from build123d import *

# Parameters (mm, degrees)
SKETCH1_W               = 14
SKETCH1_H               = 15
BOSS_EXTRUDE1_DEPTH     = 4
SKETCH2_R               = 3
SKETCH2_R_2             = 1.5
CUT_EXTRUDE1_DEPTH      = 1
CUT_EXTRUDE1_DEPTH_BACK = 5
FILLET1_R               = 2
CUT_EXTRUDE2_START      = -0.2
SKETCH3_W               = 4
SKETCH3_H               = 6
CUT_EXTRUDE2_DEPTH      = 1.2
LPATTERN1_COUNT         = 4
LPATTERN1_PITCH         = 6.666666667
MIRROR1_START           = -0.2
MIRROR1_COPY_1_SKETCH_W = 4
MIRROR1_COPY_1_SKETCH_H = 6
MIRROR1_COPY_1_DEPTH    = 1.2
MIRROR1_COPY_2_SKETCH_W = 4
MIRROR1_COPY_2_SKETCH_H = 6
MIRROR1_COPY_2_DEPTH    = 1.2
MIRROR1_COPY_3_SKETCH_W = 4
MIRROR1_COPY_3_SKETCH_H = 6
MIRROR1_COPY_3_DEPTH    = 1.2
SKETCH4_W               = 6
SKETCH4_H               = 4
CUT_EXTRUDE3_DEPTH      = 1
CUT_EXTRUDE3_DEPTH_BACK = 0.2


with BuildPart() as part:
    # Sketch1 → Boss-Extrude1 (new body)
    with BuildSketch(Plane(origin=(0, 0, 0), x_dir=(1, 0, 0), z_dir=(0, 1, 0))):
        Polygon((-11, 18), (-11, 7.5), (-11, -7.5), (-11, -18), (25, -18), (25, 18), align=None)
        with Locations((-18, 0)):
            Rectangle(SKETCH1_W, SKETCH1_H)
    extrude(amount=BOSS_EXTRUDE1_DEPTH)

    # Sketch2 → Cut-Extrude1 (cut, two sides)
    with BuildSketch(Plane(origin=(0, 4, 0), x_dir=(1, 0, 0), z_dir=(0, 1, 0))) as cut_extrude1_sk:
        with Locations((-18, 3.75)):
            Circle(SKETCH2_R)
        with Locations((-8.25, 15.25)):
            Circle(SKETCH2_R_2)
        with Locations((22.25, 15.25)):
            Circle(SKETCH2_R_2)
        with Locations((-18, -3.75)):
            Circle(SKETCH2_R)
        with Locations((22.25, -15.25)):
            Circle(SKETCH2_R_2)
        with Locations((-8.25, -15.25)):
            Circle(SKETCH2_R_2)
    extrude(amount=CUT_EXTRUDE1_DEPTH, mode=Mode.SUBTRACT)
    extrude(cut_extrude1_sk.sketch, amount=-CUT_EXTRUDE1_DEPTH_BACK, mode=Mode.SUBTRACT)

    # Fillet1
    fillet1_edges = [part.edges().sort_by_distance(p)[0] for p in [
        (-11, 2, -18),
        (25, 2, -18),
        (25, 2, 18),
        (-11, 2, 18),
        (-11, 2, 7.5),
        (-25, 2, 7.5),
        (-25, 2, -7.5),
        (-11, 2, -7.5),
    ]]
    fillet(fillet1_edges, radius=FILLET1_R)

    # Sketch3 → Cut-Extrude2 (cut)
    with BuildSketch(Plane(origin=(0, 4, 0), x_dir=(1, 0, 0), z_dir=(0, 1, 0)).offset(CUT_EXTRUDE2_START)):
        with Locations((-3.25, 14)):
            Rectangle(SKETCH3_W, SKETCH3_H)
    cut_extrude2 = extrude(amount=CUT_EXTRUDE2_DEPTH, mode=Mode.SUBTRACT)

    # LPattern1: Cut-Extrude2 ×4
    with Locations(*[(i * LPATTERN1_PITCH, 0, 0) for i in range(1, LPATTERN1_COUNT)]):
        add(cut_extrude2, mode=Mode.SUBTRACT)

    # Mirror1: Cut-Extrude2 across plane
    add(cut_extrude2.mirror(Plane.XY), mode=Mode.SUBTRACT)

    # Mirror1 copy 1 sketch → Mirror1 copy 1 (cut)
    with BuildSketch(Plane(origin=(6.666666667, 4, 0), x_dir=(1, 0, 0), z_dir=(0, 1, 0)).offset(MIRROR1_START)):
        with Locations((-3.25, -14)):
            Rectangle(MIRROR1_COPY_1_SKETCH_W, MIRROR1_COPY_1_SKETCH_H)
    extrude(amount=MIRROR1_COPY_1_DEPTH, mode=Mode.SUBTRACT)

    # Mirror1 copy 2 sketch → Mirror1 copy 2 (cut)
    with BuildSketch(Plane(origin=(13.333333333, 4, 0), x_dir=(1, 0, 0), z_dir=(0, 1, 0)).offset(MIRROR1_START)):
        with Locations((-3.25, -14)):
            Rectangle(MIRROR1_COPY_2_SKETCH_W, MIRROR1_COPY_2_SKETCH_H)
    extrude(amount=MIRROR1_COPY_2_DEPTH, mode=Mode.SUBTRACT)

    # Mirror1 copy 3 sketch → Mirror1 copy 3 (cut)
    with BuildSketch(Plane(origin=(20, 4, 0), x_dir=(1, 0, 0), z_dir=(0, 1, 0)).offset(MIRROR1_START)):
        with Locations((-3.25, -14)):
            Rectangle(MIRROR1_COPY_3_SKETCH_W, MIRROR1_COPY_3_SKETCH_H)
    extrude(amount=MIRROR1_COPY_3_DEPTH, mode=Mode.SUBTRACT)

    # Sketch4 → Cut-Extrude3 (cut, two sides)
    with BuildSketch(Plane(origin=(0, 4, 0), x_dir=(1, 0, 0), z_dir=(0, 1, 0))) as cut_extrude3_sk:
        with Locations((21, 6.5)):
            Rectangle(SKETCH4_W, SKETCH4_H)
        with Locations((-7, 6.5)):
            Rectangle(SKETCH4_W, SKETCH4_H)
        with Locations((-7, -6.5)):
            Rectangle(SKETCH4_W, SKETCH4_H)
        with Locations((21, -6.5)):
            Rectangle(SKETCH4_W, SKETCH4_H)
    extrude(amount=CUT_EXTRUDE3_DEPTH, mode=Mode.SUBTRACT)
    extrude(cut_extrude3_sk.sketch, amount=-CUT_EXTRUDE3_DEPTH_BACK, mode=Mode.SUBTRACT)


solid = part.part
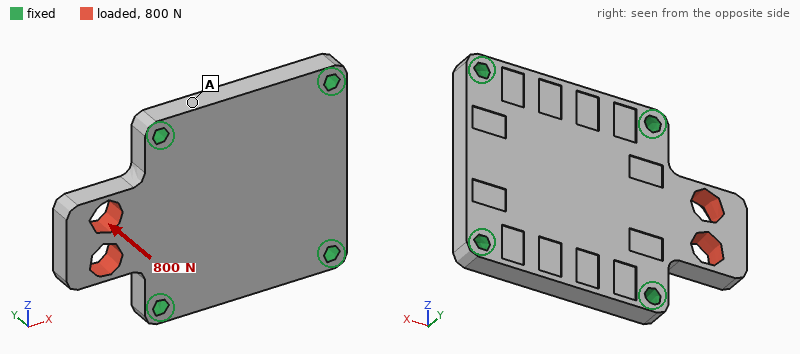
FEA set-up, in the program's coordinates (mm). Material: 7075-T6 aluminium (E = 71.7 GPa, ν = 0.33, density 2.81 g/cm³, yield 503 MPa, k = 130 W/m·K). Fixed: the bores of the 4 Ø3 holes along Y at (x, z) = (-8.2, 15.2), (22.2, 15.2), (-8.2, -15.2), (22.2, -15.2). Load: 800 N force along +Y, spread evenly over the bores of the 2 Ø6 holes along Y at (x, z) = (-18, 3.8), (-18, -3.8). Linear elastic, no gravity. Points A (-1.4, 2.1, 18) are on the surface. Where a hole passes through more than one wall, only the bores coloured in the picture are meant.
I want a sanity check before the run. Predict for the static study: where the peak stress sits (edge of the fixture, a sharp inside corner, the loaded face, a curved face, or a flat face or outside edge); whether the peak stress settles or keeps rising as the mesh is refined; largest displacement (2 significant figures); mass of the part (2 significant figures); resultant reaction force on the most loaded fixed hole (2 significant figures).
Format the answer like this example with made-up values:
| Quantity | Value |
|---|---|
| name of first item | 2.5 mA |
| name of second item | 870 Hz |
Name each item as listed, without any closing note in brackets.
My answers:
| Quantity | Value |
|---|---|
| where the peak stress sits | edge of the fixture |
| whether the peak stress settles or keeps rising as the mesh is refined | keeps rising |
| largest displacement | 0.26 mm |
| mass of the part | 16 g |
| resultant reaction force on the most loaded fixed hole | 500 N |
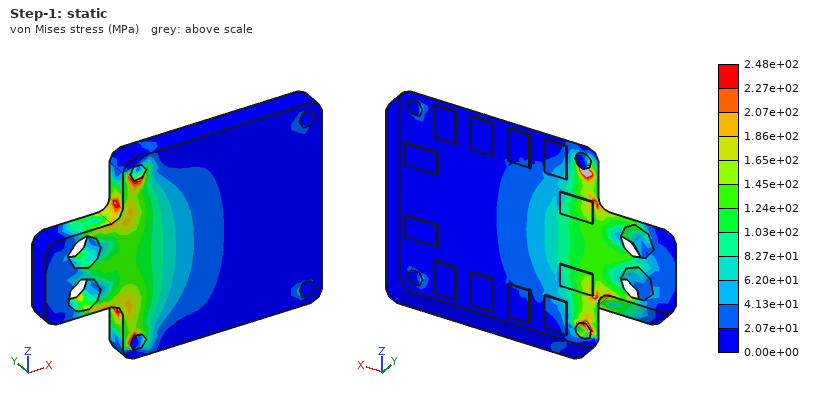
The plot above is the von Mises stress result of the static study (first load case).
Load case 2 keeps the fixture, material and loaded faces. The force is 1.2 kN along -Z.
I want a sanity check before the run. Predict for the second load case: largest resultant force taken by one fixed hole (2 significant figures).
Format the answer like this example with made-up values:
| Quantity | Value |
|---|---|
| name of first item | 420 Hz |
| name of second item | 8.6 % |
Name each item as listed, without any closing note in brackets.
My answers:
| Quantity | Value |
|---|---|
| largest resultant force taken by one fixed hole | 670 N |
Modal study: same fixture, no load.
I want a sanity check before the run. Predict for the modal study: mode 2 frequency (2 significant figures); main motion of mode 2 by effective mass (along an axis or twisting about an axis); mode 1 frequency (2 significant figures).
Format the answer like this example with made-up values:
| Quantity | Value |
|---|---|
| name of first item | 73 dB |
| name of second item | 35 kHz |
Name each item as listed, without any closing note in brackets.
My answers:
| Quantity | Value |
|---|---|
| mode 2 frequency | 14 kHz |
| main motion of mode 2 by effective mass | along Y |
| mode 1 frequency | 7600 Hz |
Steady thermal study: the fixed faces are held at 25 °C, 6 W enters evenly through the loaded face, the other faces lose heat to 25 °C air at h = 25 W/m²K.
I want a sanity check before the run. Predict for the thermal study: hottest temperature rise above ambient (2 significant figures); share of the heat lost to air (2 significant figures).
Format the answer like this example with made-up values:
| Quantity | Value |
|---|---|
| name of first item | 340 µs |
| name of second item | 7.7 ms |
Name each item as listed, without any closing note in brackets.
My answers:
| Quantity | Value |
|---|---|
| hottest temperature rise above ambient | 17 K |
| share of the heat lost to air | 4.4 % |
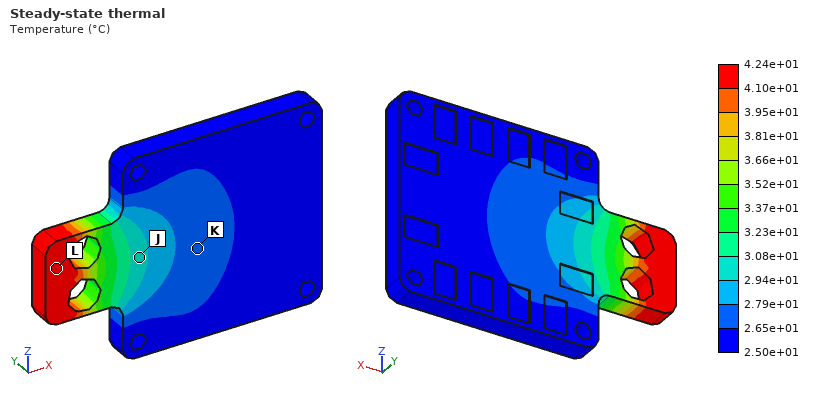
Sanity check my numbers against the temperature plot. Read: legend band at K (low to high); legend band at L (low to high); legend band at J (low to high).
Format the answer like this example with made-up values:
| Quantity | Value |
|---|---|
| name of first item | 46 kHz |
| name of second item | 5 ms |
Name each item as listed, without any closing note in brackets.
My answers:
| Quantity | Value |
|---|---|
| legend band at K | 2.65e+01 to 2.79e+01 °C |
| legend band at L | 4.10e+01 to 4.24e+01 °C |
| legend band at J | 2.94e+01 to 3.08e+01 °C |
